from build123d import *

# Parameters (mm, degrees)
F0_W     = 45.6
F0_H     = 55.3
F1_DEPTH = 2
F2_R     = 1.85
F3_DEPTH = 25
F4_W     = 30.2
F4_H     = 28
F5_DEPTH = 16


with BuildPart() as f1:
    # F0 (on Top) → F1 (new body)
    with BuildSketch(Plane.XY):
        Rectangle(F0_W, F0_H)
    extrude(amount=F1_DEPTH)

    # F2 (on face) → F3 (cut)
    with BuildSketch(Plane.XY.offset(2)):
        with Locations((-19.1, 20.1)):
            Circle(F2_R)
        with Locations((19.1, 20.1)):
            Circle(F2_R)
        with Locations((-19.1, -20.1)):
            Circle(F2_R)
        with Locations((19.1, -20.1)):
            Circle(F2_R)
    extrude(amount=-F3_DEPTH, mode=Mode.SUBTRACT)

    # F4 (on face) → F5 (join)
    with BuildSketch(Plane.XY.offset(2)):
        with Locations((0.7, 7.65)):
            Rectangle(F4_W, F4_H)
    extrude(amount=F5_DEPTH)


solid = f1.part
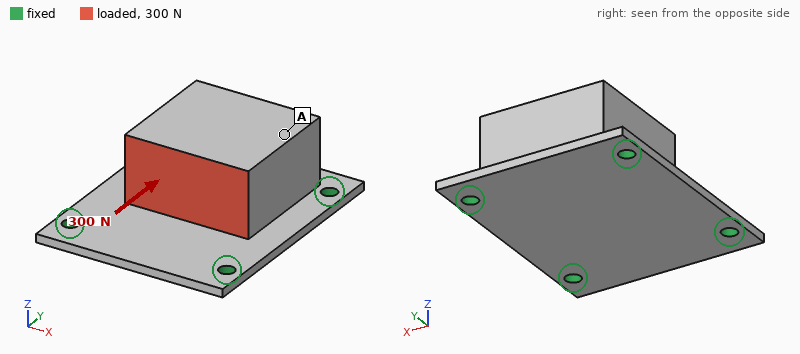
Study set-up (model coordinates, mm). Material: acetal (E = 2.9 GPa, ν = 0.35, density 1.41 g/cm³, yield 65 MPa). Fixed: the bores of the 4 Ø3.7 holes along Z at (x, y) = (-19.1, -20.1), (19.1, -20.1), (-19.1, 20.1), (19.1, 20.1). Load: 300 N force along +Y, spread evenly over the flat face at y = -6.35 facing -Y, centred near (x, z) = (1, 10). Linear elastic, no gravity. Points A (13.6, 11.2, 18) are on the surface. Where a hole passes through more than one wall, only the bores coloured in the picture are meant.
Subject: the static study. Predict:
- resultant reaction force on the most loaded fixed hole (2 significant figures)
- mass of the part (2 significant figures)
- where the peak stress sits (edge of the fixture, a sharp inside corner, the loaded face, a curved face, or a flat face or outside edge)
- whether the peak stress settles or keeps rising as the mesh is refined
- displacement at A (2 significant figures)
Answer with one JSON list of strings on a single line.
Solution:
["100 N", "26 g", "edge of the fixture", "keeps rising", "0.23 mm"]
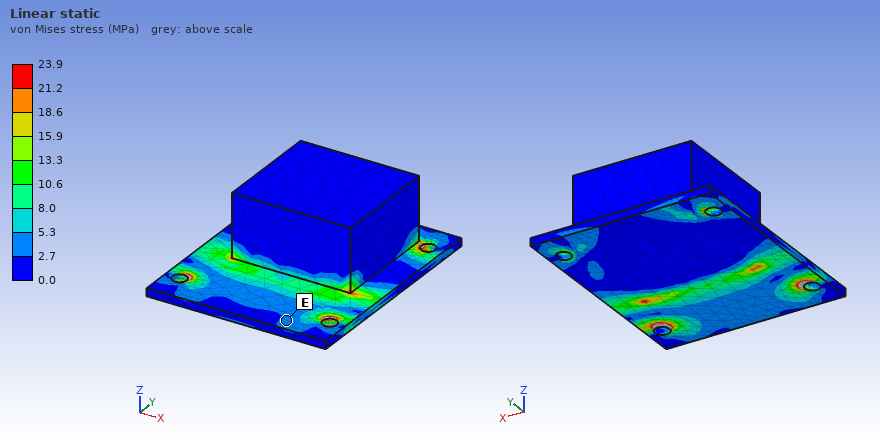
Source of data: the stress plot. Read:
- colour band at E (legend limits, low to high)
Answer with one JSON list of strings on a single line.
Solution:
["2.7 to 5.3 MPa"]
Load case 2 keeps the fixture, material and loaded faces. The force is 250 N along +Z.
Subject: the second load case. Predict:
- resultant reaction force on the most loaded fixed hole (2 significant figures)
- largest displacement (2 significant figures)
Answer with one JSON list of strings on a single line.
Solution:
["91 N", "0.84 mm"]
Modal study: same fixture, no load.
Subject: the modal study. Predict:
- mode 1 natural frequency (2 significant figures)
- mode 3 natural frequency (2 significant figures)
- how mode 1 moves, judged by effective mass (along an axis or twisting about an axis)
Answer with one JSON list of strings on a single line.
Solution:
["910 Hz", "2600 Hz", "along Z"]
